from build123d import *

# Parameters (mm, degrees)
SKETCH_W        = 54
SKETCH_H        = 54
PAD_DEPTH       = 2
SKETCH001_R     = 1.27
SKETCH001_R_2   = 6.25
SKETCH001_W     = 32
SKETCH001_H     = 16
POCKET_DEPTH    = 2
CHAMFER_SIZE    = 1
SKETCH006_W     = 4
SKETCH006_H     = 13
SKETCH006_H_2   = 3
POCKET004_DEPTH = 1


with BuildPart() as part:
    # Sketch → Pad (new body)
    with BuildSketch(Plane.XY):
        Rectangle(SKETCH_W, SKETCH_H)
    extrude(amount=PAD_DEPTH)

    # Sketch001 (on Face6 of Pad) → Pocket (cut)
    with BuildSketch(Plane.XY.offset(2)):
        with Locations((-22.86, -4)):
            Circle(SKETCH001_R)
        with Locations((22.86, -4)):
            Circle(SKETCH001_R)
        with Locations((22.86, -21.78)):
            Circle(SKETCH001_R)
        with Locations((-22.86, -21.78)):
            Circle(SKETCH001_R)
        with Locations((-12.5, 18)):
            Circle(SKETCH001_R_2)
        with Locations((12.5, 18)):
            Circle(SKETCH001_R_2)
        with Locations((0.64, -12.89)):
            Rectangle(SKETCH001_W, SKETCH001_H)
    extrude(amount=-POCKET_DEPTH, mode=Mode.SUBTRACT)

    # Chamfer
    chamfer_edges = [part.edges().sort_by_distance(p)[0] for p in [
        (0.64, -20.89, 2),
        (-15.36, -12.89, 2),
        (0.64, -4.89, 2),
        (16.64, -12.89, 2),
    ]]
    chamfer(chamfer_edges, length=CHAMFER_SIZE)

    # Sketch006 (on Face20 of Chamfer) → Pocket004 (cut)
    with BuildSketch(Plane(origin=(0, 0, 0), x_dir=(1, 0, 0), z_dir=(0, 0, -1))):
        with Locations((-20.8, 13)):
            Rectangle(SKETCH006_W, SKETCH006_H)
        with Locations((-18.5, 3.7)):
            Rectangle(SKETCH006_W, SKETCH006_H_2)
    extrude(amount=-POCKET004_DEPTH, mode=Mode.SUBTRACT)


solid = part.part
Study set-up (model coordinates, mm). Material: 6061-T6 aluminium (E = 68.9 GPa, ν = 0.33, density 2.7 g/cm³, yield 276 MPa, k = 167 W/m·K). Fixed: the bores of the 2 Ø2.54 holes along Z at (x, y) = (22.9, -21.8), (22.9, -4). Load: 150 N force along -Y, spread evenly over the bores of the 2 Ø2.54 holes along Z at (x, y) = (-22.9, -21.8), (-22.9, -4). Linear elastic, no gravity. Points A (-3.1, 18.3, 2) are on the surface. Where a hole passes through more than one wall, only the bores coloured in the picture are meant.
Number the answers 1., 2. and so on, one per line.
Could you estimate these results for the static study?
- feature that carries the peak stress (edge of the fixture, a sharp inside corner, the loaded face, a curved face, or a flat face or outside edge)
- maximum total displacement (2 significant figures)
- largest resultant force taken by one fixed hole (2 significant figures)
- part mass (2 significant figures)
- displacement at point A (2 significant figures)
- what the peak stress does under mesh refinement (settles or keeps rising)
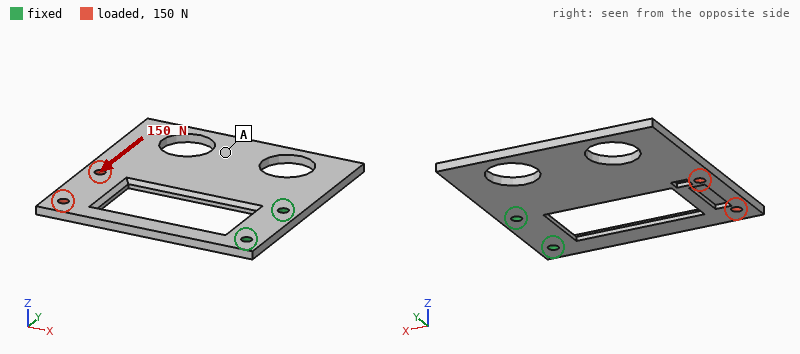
1. edge of the fixture
2. 0.14 mm
3. 320 N
4. 11 g
5. 0.080 mm
6. keeps rising
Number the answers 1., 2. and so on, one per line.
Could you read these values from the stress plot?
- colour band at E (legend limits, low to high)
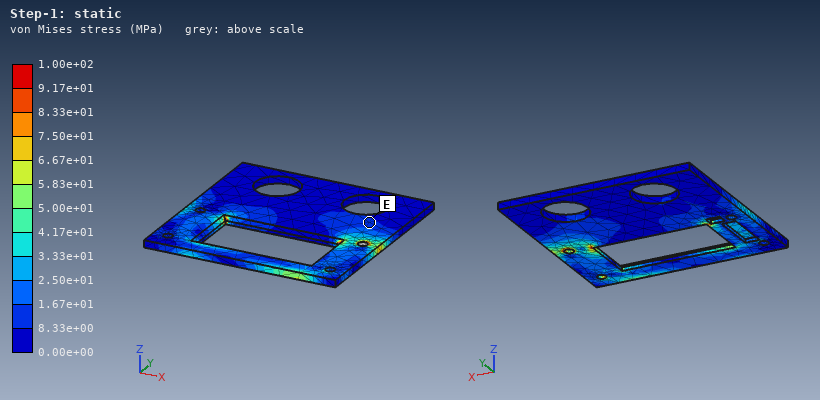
1. 8.33e+00 to 1.67e+01 MPa
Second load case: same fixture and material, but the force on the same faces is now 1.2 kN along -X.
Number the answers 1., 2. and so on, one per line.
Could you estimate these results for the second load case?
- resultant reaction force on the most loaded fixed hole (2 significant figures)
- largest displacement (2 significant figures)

1. 600 N
2. 48 µm
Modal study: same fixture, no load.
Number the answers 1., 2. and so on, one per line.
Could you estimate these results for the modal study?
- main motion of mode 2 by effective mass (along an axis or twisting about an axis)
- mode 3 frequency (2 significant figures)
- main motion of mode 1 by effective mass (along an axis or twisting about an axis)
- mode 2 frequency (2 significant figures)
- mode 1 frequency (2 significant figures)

1. twisting about X
2. 2100 Hz
3. along Z
4. 950 Hz
5. 450 Hz
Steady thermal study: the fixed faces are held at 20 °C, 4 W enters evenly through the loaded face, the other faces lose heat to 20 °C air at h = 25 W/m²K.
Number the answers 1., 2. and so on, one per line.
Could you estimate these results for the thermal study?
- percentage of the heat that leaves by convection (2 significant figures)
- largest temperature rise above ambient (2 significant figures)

1. 30 %
2. 24 K
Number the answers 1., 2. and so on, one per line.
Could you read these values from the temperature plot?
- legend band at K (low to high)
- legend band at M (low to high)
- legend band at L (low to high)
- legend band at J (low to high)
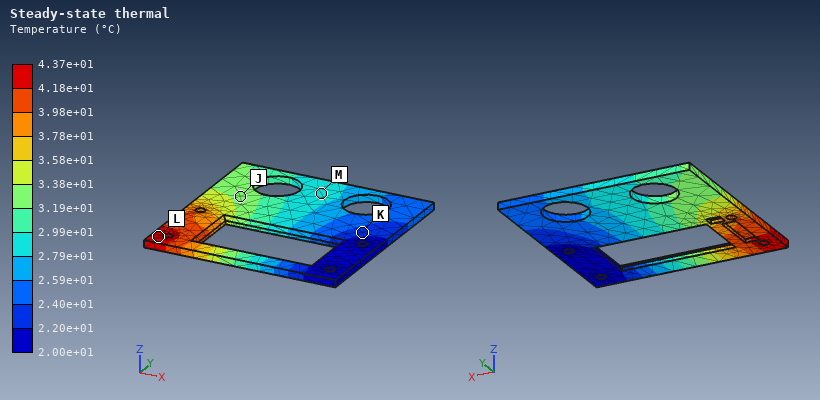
1. 2.20e+01 to 2.40e+01 °C
2. 2.79e+01 to 2.99e+01 °C
3. 4.18e+01 to 4.37e+01 °C
4. 3.19e+01 to 3.38e+01 °C
